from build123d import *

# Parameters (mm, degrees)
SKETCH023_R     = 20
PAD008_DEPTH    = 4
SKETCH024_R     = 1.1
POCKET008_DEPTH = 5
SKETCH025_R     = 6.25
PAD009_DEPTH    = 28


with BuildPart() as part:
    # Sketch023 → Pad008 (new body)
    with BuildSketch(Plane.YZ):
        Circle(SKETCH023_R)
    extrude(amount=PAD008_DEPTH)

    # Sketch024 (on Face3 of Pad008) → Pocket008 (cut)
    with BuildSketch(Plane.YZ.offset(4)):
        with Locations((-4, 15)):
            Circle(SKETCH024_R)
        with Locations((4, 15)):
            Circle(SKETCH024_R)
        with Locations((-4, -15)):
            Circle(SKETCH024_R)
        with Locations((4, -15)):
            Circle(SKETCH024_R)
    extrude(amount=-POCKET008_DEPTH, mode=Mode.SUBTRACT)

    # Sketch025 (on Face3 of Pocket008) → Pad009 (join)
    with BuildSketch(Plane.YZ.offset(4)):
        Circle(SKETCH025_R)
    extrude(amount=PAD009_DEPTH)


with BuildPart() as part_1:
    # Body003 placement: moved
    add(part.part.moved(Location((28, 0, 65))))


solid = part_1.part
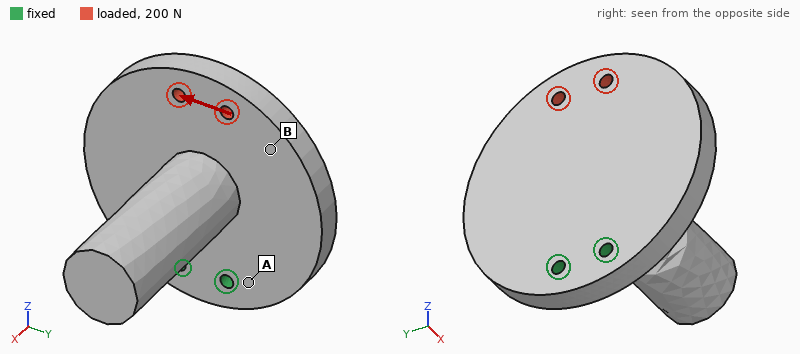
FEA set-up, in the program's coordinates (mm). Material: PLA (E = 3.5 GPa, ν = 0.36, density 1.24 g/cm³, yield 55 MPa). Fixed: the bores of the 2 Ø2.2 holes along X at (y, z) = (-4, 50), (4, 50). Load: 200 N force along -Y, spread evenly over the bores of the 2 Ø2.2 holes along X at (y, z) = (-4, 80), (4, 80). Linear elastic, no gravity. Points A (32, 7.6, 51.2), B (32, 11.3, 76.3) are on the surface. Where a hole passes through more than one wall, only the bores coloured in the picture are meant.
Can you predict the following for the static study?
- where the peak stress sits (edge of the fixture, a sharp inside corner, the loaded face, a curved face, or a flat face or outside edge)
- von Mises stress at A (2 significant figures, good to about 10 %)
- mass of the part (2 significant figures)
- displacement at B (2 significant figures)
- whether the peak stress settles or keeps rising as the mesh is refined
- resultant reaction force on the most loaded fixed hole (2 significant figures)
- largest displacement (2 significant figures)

edge of the fixture
10 MPa
10 g
0.30 mm
keeps rising
620 N
0.38 mm
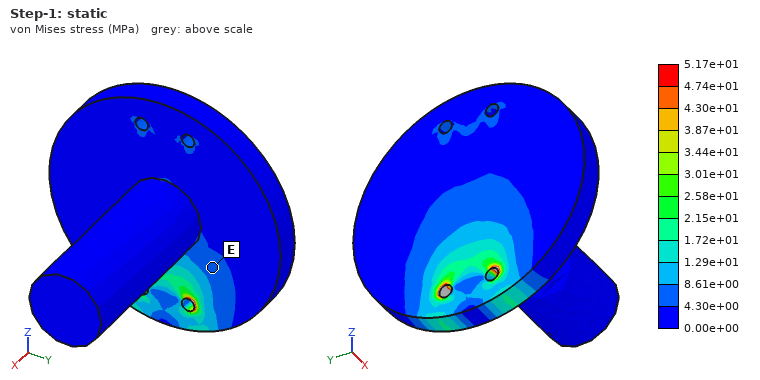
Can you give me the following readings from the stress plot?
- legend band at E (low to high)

4.30e+00 to 8.61e+00 MPa
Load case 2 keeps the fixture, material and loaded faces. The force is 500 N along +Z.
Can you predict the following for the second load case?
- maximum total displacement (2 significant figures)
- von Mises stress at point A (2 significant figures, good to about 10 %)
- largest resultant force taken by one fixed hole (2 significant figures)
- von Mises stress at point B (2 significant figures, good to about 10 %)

70 µm
3.7 MPa
250 N
1.8 MPa
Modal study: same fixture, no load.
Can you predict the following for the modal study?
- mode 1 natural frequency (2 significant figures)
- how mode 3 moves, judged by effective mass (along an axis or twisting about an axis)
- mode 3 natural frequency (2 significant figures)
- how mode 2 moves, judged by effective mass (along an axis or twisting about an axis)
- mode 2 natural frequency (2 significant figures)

580 Hz
along Y
2200 Hz
along Y
1000 Hz
